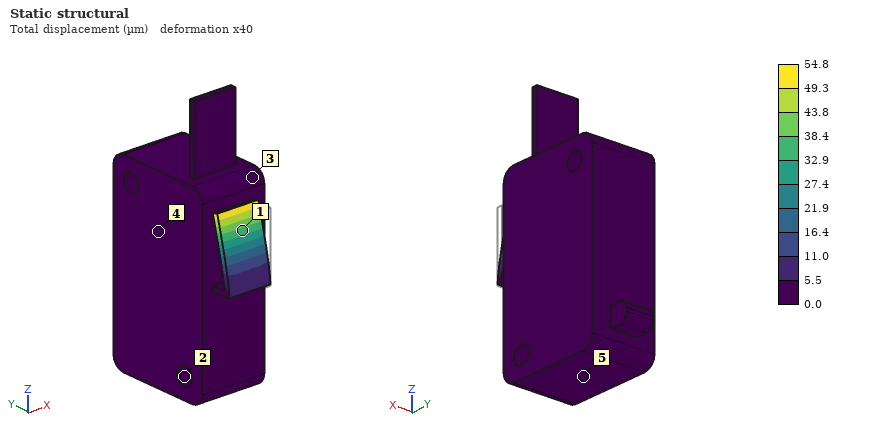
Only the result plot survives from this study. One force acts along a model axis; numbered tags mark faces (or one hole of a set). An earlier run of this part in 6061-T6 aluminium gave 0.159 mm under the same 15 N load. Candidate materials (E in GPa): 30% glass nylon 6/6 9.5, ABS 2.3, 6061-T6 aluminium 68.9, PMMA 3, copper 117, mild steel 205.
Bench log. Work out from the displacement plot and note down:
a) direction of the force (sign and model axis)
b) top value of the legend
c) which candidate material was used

+Y
54.8 µm
mild steel
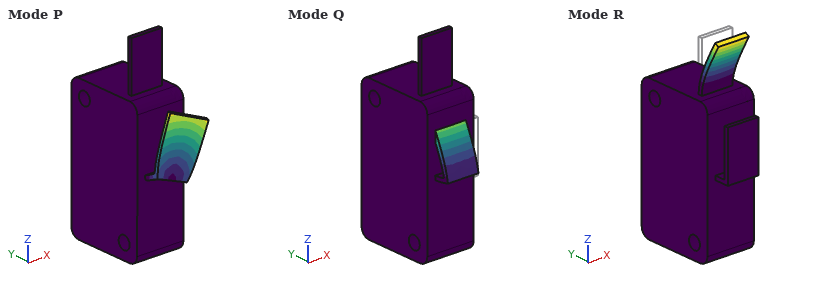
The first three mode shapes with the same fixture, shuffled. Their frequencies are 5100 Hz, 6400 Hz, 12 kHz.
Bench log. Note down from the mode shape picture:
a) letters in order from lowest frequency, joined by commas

Q, R, P
